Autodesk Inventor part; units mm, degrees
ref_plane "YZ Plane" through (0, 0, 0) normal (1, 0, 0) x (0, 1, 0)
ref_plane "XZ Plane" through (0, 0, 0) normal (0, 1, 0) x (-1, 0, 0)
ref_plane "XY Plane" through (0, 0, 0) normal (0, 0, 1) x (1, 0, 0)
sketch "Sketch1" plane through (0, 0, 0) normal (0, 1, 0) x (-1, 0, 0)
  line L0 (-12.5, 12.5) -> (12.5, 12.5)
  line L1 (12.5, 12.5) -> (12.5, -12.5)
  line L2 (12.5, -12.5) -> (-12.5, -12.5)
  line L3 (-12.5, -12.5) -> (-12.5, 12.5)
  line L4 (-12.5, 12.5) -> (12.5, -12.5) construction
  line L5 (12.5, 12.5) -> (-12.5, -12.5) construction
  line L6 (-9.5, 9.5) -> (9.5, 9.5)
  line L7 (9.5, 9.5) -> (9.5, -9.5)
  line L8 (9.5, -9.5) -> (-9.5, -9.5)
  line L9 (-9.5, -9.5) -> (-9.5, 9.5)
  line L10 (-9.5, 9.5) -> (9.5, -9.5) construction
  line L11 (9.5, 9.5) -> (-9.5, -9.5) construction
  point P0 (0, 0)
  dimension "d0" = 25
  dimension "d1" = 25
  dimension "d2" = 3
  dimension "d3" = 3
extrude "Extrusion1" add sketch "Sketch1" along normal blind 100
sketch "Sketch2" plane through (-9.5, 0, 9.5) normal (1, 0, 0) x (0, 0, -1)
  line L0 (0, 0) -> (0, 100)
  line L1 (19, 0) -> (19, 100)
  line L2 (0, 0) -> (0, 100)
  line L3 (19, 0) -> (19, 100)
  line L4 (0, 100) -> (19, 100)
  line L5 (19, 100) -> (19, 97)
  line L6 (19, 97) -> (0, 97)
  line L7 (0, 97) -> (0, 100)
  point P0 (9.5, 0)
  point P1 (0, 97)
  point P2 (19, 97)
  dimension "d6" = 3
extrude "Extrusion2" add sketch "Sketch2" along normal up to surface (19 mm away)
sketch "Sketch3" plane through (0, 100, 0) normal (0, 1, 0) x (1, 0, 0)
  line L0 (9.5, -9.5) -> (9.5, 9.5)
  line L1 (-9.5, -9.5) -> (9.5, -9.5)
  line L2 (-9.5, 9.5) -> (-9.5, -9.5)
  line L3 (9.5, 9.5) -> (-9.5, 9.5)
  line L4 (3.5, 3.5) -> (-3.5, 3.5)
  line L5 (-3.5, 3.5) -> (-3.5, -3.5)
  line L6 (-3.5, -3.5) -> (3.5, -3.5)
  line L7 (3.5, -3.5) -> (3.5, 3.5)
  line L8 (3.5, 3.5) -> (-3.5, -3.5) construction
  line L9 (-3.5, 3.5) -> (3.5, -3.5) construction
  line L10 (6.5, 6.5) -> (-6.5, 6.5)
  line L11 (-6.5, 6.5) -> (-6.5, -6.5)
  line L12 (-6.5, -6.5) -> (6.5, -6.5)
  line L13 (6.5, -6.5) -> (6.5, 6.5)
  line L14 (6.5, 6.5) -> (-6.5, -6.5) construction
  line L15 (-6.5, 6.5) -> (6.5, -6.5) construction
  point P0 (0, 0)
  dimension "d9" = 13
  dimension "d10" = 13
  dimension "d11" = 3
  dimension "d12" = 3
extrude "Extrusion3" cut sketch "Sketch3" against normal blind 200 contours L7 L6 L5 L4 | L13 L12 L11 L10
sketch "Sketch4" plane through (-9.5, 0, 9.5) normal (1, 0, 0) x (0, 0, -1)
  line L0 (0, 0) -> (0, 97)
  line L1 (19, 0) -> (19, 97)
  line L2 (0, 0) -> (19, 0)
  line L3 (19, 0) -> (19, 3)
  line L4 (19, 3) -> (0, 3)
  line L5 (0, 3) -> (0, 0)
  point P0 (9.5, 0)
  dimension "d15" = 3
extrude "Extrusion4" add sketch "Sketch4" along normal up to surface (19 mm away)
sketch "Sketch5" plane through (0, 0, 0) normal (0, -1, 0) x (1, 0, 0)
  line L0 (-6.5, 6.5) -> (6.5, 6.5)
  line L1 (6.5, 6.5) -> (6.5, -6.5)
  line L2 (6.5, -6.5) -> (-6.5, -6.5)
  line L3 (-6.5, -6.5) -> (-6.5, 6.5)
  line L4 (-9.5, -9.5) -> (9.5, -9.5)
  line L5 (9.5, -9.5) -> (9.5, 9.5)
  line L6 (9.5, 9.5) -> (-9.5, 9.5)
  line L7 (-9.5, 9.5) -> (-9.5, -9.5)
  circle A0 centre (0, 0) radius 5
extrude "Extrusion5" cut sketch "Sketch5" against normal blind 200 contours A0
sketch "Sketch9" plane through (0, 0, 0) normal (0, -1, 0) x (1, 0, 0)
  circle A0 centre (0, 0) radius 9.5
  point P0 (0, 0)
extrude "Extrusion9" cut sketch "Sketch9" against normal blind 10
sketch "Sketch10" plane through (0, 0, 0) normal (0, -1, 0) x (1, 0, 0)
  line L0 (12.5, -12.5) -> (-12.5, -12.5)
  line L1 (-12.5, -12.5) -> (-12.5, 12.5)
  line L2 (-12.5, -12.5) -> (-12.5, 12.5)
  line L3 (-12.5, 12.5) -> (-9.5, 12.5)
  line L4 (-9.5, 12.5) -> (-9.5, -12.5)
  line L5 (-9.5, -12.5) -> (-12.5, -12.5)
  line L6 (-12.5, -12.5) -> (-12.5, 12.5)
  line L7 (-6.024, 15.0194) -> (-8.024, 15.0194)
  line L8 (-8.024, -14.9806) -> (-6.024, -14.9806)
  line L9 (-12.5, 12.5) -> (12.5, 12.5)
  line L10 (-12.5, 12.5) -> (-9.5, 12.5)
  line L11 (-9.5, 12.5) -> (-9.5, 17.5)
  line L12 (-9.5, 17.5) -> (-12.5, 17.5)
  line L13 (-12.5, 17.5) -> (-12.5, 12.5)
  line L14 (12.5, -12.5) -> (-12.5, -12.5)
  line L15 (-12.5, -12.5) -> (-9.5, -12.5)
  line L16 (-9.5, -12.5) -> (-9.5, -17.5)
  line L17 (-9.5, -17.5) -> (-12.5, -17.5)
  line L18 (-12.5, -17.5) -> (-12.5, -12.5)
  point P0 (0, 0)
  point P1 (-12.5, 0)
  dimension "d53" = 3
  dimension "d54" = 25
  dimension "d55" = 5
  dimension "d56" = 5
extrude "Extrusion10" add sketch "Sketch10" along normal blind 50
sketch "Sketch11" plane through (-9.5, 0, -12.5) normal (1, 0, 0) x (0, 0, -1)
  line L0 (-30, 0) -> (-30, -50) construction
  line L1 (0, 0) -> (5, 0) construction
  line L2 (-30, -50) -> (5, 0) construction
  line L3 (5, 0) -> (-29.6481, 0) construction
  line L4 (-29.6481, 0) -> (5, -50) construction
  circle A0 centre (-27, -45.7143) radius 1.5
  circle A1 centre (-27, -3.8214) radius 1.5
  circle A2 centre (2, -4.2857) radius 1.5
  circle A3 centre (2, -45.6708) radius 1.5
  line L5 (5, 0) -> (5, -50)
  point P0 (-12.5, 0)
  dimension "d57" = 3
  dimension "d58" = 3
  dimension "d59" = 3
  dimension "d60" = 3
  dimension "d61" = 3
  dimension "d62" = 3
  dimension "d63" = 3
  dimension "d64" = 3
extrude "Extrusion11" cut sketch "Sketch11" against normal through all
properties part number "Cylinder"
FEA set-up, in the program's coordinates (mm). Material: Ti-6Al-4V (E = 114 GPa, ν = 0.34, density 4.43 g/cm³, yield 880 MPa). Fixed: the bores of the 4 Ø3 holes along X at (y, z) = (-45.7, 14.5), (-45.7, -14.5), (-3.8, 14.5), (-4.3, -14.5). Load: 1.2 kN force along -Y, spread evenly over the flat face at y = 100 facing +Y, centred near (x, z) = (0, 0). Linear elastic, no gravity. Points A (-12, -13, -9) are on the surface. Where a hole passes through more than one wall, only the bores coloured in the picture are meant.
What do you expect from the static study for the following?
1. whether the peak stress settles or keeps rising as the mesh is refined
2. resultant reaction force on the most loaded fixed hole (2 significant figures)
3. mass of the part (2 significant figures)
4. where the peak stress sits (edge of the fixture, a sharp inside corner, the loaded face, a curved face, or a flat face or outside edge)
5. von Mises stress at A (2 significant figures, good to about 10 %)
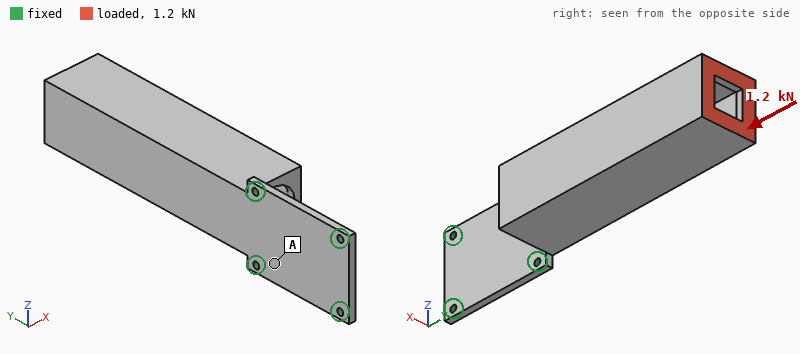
keeps rising
490 N
140 g
edge of the fixture
34 MPa
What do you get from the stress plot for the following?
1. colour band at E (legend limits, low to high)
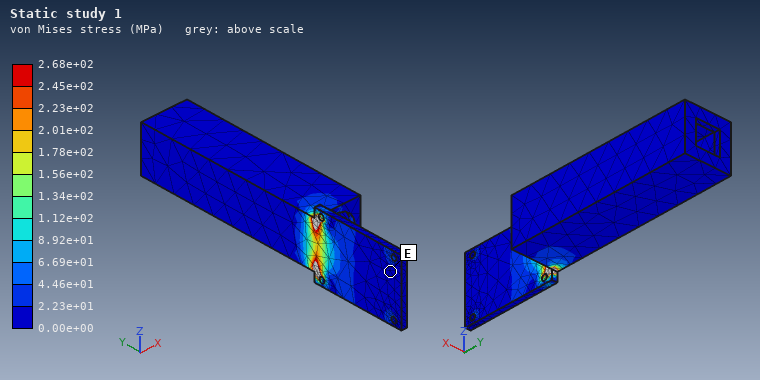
0.00e+00 to 2.23e+01 MPa
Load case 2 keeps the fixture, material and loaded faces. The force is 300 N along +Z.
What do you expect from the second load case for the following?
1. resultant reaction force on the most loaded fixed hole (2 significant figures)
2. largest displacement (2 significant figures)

1.0 kN
0.14 mm
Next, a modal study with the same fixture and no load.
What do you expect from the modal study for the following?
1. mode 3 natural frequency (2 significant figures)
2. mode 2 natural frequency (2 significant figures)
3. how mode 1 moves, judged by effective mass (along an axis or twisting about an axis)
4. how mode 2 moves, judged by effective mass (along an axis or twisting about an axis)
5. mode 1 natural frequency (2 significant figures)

2500 Hz
1200 Hz
along X
along Z
210 Hz
